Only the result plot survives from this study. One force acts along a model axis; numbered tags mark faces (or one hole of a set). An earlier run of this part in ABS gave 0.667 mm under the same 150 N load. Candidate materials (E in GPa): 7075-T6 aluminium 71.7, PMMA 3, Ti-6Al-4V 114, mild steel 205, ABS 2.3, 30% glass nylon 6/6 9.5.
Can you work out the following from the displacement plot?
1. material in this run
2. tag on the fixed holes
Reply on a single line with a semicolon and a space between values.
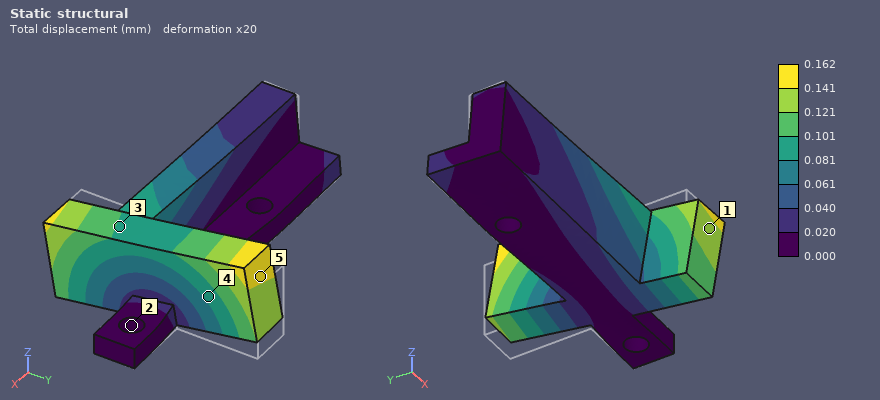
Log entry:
30% glass nylon 6/6; 2
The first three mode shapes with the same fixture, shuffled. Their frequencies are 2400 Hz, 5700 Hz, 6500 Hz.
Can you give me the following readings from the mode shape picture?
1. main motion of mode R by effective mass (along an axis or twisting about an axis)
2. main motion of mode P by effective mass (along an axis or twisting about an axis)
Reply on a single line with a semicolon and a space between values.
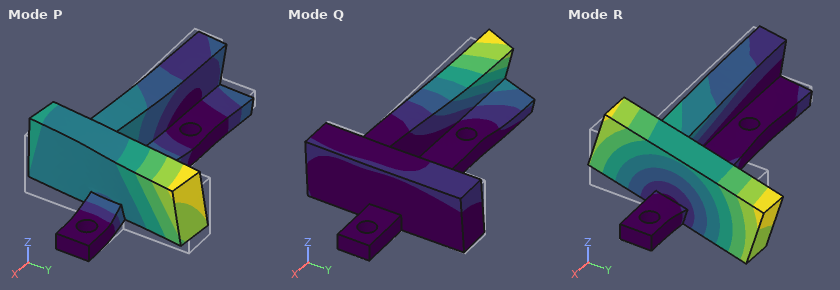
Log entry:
along Y; along Z
